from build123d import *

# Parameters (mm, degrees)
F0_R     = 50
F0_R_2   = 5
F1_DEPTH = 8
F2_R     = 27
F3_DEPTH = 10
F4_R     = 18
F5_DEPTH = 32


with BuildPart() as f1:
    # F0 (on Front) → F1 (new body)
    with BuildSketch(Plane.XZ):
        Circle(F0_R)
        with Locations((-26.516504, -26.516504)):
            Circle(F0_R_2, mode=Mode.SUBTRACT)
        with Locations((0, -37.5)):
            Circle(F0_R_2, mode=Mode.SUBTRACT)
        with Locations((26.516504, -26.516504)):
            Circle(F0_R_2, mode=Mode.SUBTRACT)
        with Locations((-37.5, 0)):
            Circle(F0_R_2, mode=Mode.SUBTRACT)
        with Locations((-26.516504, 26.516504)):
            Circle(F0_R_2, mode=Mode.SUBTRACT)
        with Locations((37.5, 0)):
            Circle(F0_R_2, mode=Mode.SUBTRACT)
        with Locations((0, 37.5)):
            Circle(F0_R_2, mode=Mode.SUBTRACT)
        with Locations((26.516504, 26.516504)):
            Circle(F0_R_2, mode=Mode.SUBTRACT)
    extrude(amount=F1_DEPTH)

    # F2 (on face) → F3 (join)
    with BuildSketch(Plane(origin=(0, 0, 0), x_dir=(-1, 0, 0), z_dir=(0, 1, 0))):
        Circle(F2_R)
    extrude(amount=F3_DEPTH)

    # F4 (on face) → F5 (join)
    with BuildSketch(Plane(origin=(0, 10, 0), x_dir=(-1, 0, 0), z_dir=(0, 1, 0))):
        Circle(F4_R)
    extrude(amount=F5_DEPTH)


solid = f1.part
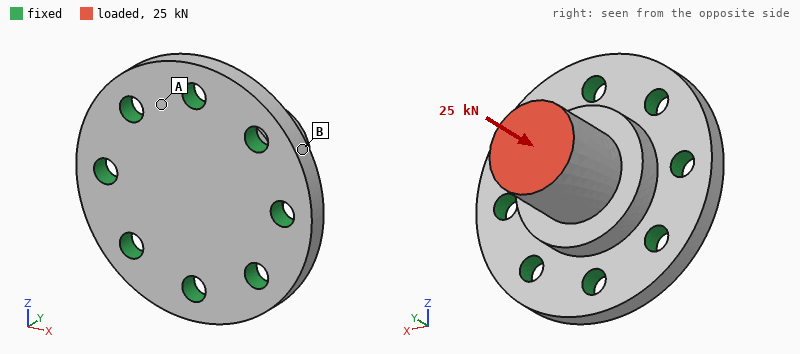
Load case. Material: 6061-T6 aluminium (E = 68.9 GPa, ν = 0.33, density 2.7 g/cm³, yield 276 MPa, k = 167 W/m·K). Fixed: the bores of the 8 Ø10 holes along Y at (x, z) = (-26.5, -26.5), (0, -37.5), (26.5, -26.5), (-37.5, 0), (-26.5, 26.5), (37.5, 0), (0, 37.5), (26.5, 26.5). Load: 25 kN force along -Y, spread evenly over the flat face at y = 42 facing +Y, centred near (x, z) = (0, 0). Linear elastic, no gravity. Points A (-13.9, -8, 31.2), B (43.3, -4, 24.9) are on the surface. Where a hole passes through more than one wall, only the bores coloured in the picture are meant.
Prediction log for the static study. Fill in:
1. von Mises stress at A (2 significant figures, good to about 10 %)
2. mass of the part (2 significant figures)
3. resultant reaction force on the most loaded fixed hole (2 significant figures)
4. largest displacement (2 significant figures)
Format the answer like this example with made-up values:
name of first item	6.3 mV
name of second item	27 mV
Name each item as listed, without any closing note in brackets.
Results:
von Mises stress at A	24 MPa
mass of the part	310 g
resultant reaction force on the most loaded fixed hole	3.9 kN
largest displacement	33 µm
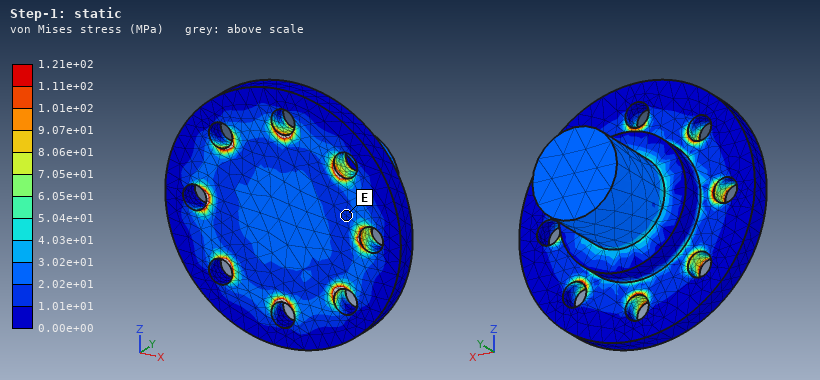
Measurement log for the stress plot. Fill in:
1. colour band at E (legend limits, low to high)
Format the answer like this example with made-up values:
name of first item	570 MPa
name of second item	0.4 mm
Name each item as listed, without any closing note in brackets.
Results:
colour band at E	1.01e+01 to 2.02e+01 MPa
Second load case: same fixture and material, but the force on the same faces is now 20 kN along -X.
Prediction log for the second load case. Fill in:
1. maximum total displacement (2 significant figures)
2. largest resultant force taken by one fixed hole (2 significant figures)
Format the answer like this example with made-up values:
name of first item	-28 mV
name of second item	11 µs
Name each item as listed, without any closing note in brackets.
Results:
maximum total displacement	0.17 mm
largest resultant force taken by one fixed hole	9.0 kN
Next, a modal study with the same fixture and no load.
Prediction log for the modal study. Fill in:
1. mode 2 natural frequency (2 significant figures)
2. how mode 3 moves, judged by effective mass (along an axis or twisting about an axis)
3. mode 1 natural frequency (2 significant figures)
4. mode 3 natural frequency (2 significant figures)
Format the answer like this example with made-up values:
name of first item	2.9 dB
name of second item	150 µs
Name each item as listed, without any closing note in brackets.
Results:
mode 2 natural frequency	9300 Hz
how mode 3 moves, judged by effective mass	along Y
mode 1 natural frequency	9200 Hz
mode 3 natural frequency	12 kHz
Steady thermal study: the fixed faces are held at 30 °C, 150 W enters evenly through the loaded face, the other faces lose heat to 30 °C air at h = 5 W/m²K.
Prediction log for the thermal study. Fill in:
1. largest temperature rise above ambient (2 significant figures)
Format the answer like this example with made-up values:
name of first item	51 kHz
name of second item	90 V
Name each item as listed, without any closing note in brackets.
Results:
largest temperature rise above ambient	44 K
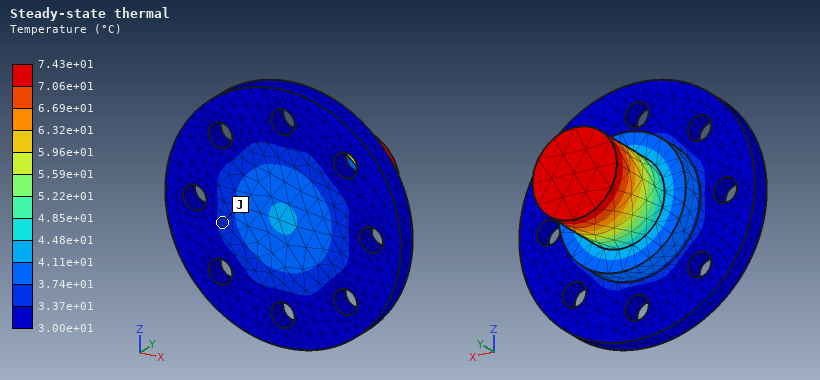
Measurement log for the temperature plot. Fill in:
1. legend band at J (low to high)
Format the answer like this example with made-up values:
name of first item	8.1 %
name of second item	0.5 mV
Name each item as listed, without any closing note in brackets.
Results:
legend band at J	3.37e+01 to 3.74e+01 °C
